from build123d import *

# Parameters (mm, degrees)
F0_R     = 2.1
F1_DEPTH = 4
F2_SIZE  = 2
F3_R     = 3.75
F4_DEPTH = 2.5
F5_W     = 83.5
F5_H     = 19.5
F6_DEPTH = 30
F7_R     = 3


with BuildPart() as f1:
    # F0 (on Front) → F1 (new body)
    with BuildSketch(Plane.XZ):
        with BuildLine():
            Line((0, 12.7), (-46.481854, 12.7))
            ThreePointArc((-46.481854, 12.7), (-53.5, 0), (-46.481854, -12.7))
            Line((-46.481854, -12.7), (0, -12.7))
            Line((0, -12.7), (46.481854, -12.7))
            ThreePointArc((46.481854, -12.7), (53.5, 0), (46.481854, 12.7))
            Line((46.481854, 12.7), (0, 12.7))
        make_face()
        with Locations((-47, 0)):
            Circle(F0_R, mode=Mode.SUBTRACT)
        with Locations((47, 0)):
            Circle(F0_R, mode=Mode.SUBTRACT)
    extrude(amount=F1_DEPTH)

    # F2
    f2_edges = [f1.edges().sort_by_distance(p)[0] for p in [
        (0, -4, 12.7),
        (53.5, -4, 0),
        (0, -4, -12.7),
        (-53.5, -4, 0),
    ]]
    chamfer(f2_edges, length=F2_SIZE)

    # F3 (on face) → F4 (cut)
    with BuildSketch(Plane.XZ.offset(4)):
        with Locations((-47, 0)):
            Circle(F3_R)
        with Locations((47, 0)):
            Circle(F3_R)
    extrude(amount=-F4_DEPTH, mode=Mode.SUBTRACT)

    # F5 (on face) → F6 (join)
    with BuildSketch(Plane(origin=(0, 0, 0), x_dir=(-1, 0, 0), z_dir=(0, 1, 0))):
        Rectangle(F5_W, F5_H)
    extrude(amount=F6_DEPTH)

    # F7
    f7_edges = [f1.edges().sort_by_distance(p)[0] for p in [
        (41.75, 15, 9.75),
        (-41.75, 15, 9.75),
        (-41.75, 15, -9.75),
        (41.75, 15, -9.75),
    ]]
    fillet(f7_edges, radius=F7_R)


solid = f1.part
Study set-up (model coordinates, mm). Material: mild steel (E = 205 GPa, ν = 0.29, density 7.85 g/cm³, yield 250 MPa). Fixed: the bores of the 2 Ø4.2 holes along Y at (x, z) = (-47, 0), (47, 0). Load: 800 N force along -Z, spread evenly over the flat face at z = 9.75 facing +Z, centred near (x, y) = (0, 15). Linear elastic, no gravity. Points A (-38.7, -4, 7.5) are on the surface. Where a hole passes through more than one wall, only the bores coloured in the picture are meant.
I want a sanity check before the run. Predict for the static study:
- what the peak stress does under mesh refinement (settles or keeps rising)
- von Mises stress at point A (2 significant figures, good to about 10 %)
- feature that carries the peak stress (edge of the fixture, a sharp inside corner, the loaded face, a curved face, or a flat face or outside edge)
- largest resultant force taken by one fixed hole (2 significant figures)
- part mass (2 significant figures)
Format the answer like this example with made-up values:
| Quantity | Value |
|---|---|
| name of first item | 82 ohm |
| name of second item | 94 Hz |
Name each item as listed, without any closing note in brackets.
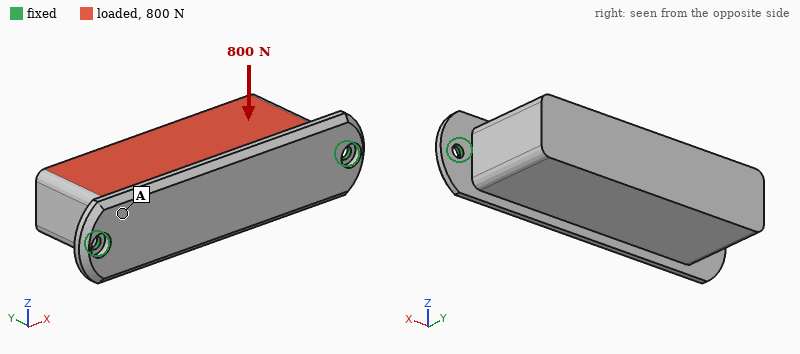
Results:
| Quantity | Value |
|---|---|
| what the peak stress does under mesh refinement | keeps rising |
| von Mises stress at point A | 39 MPa |
| feature that carries the peak stress | edge of the fixture |
| largest resultant force taken by one fixed hole | 400 N |
| part mass | 460 g |
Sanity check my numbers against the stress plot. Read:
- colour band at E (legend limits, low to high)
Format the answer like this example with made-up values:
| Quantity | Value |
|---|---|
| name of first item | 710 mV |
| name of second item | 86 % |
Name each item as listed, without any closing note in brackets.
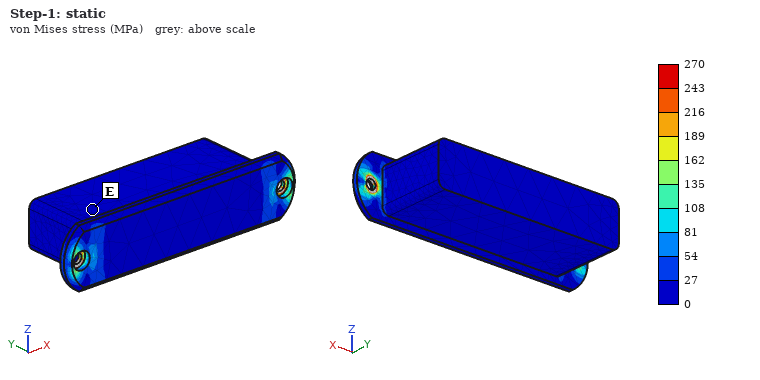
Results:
| Quantity | Value |
|---|---|
| colour band at E | 0 to 27 MPa |
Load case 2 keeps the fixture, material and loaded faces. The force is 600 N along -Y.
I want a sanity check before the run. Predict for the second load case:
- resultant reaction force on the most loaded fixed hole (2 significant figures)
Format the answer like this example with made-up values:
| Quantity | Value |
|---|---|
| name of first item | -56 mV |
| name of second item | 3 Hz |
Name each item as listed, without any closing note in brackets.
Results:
| Quantity | Value |
|---|---|
| resultant reaction force on the most loaded fixed hole | 300 N |
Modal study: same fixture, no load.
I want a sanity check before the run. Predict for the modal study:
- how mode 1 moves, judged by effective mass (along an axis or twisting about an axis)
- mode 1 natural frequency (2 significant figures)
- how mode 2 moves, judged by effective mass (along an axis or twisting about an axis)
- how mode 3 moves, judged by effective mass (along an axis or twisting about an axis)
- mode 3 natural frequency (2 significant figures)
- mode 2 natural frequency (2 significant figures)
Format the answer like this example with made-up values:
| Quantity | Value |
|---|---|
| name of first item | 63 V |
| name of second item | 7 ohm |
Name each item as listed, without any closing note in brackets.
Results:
| Quantity | Value |
|---|---|
| how mode 1 moves, judged by effective mass | along Z |
| mode 1 natural frequency | 800 Hz |
| how mode 2 moves, judged by effective mass | along Y |
| how mode 3 moves, judged by effective mass | along X |
| mode 3 natural frequency | 5300 Hz |
| mode 2 natural frequency | 3700 Hz |
